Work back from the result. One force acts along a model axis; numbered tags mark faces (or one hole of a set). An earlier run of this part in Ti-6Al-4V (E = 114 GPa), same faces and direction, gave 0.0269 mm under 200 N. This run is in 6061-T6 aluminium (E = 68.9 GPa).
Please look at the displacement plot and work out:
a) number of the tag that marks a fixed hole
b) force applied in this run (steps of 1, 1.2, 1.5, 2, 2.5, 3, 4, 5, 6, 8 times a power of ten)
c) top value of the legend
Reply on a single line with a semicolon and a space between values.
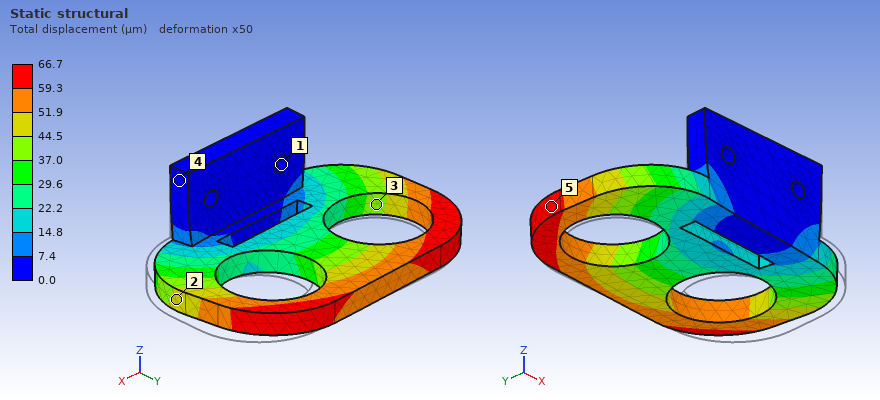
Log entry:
1; 300 N; 66.7 µm
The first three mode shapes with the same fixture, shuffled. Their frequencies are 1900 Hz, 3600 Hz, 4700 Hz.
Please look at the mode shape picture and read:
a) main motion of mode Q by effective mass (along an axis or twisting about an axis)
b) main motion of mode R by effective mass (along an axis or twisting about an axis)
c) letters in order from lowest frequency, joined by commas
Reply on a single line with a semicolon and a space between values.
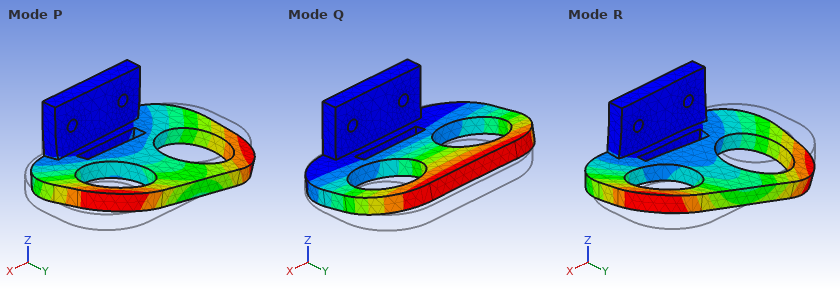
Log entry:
along Z; along X; Q, P, R
